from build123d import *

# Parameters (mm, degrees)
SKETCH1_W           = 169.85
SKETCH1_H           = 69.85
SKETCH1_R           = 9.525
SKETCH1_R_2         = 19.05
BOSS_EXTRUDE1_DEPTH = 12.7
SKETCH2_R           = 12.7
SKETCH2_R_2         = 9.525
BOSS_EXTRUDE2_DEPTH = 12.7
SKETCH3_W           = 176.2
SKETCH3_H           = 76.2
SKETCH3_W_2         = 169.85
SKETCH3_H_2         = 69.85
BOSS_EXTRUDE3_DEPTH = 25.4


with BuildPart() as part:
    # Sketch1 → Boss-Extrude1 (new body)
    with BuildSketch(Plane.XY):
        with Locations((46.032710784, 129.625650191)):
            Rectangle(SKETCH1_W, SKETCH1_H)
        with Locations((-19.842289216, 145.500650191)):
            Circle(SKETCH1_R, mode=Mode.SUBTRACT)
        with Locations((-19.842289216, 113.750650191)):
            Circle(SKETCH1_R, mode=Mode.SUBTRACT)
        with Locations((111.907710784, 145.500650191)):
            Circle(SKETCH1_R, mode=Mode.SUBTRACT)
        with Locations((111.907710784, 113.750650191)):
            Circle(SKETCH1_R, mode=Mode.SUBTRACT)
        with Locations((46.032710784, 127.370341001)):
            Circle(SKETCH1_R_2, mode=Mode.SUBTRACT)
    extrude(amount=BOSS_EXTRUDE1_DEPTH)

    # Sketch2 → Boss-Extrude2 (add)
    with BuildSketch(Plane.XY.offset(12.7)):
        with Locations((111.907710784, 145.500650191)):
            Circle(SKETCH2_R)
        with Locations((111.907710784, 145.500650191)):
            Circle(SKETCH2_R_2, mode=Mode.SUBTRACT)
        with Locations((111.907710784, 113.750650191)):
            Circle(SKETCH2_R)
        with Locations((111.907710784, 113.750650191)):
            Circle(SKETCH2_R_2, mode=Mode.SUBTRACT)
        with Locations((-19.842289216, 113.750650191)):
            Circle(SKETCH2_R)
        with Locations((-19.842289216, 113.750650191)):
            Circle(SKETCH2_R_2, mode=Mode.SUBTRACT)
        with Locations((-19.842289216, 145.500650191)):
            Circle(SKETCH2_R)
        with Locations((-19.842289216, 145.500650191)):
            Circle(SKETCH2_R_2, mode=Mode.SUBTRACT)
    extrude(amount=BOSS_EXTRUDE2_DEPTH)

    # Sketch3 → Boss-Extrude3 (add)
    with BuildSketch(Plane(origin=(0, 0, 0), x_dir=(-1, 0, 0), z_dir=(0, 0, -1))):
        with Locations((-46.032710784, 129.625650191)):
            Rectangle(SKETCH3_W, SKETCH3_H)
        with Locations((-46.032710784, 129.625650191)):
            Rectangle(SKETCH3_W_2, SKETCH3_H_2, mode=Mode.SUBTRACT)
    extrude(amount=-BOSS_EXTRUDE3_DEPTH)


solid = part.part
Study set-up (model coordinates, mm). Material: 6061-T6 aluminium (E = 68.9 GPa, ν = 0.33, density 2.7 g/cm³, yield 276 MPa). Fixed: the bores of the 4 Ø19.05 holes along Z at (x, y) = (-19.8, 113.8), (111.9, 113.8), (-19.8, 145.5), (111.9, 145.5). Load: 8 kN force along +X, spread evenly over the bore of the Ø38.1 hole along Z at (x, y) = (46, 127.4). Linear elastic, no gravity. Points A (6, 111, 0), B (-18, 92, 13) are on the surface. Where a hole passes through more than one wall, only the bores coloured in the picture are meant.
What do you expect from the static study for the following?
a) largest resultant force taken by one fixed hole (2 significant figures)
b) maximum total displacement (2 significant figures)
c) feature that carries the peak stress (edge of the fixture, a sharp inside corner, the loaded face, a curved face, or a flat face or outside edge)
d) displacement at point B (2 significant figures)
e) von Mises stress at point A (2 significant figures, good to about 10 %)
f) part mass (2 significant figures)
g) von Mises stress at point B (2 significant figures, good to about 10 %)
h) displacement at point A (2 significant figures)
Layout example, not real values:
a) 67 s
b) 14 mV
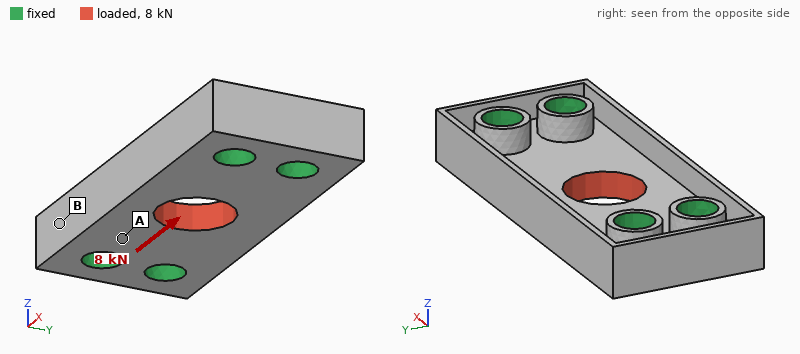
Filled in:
a) 2.1 kN
b) 4.2 µm
c) the loaded face
d) 0.94 µm
e) 5.1 MPa
f) 470 g
g) 1.8 MPa
h) 1.5 µm
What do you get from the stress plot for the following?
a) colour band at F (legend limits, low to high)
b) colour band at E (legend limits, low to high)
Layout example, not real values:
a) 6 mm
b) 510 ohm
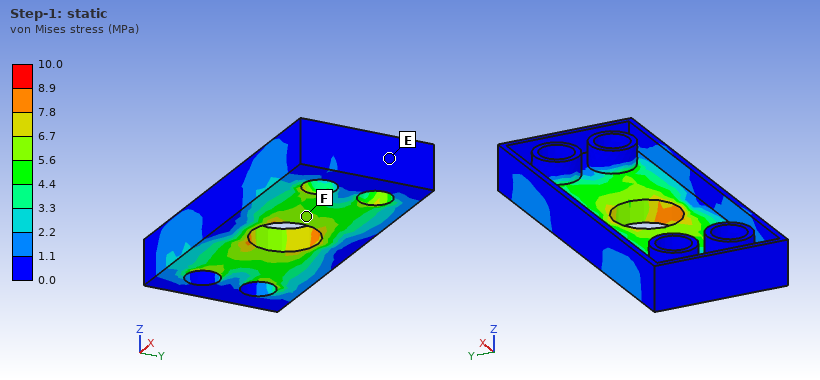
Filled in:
a) 5.6 to 6.7 MPa
b) 0.0 to 1.1 MPa
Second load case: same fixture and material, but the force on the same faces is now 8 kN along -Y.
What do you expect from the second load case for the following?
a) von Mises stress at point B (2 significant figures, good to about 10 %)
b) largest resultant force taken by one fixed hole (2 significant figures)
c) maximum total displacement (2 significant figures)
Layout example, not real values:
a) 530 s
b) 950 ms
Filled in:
a) 4.0 MPa
b) 2.7 kN
c) 15 µm
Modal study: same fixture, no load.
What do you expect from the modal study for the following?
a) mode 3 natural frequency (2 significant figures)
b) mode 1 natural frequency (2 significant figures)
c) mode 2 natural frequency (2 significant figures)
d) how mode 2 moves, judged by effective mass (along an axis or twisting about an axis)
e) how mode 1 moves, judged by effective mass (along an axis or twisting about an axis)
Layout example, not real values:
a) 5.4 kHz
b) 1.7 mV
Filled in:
a) 10 kHz
b) 5400 Hz
c) 5900 Hz
d) twisting about X
e) along Z
